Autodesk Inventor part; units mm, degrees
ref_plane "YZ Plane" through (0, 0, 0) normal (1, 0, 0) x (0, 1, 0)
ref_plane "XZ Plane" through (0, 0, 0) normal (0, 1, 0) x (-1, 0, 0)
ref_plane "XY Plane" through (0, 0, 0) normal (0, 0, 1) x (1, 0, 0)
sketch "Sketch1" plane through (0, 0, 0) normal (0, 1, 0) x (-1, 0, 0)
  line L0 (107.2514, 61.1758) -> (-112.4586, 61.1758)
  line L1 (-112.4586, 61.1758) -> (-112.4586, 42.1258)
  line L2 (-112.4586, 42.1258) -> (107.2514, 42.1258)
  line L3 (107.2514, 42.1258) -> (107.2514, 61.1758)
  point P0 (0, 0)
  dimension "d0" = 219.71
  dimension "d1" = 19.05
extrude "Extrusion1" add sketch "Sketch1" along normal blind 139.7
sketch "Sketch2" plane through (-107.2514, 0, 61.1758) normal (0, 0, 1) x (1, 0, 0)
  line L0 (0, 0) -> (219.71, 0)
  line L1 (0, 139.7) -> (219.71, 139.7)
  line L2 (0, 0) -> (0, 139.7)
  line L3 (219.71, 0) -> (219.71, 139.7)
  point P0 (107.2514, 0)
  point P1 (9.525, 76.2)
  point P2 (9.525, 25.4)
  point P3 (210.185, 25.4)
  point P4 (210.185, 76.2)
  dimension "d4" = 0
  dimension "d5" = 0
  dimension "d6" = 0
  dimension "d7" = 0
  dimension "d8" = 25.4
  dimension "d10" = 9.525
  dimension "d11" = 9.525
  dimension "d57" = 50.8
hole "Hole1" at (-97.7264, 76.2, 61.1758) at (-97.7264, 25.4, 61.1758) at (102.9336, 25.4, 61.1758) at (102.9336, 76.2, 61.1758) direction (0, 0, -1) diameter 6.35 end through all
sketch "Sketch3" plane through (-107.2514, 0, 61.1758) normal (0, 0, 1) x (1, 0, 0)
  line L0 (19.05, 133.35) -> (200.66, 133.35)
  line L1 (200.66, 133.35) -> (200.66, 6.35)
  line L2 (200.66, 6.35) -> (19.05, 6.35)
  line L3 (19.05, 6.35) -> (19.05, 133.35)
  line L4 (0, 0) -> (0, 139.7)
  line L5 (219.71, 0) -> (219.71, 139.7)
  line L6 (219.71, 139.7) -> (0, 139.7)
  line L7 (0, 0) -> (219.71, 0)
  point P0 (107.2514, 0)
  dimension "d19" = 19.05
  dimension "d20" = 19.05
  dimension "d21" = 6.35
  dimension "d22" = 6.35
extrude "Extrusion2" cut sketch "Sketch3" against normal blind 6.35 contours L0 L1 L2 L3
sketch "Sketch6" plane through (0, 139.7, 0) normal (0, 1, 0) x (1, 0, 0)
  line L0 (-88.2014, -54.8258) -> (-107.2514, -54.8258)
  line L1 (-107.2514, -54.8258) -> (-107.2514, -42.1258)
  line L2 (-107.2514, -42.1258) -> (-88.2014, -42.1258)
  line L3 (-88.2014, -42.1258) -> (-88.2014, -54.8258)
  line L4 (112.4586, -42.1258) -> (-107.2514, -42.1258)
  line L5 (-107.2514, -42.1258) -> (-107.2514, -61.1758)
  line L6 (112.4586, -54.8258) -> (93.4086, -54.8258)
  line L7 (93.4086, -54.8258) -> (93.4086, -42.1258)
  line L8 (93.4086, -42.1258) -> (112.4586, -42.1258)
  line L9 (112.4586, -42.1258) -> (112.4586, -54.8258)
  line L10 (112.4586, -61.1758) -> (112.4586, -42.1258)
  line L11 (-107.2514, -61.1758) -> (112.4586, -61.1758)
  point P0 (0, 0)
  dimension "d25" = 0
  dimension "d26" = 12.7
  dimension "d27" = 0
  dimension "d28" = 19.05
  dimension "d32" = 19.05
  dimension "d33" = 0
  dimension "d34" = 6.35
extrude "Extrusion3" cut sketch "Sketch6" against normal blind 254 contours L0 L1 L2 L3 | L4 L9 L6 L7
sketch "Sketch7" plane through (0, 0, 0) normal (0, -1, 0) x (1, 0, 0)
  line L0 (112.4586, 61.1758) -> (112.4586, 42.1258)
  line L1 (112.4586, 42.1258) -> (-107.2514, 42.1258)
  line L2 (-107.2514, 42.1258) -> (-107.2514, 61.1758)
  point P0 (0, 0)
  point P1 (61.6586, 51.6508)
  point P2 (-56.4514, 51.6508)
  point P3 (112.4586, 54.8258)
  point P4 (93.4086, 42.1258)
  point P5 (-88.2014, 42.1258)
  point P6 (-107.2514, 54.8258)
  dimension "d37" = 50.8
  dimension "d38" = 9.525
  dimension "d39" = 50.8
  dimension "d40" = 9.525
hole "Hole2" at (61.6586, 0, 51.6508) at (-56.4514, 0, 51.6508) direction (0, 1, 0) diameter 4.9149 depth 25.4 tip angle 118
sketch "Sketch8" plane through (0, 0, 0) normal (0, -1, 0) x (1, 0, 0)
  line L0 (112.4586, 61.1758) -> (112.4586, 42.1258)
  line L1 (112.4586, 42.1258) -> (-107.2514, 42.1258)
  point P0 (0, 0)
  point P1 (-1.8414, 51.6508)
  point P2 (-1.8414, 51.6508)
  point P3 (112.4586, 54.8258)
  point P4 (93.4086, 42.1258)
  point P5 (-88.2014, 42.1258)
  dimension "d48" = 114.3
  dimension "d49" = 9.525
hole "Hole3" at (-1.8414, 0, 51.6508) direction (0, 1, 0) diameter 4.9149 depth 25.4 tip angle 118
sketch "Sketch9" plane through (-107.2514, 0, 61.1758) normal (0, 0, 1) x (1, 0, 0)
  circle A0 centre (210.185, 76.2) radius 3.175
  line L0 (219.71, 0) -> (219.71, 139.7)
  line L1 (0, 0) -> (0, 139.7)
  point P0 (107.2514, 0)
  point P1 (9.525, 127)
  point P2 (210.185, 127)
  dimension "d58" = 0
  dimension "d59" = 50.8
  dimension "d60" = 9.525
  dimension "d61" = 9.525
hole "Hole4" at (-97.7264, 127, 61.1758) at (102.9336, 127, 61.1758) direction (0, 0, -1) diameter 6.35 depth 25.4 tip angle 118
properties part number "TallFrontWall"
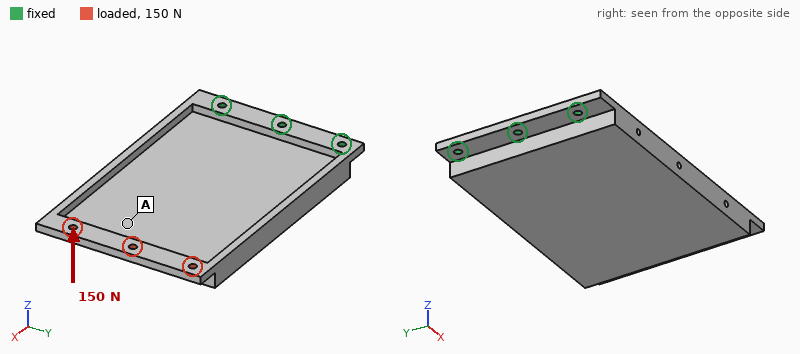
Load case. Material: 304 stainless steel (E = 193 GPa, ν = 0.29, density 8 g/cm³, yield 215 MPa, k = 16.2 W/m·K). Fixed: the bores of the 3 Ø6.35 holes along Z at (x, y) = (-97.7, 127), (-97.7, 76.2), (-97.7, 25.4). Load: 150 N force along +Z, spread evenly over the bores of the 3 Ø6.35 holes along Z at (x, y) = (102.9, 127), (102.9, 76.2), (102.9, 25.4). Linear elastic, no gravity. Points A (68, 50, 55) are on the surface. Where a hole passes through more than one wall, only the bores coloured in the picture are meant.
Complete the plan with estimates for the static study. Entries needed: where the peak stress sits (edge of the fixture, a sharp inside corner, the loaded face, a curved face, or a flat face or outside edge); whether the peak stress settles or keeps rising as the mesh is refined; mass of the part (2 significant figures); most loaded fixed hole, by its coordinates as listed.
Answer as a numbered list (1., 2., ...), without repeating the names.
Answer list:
1. a sharp inside corner
2. keeps rising
3. 2.9 kg
4. (-97.7, 76.2)
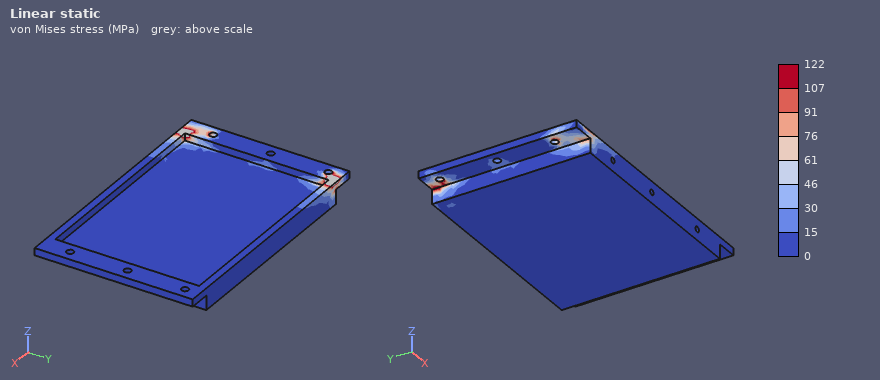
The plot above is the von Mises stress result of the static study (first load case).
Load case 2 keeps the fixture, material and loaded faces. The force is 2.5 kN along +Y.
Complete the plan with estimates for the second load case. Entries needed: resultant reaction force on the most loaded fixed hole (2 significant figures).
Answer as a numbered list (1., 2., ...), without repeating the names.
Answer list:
1. 4.8 kN
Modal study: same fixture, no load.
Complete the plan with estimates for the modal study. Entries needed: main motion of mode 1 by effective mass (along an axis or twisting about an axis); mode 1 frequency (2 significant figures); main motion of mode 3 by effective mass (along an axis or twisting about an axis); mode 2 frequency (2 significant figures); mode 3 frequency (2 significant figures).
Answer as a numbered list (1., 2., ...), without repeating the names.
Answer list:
1. along Z
2. 67 Hz
3. along Y
4. 620 Hz
5. 1200 Hz
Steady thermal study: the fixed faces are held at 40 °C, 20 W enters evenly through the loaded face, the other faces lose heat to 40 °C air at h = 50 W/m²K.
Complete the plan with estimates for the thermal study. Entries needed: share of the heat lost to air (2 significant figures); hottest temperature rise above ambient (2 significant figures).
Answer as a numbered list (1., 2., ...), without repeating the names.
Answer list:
1. 100 %
2. 49 K
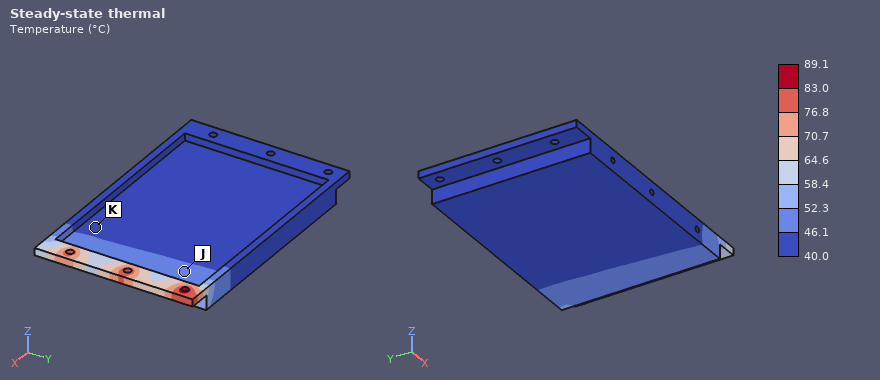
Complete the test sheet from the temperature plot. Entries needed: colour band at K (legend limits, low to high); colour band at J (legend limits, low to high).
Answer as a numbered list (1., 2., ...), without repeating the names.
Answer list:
1. 40.0 to 46.1 °C
2. 46.1 to 52.3 °C
